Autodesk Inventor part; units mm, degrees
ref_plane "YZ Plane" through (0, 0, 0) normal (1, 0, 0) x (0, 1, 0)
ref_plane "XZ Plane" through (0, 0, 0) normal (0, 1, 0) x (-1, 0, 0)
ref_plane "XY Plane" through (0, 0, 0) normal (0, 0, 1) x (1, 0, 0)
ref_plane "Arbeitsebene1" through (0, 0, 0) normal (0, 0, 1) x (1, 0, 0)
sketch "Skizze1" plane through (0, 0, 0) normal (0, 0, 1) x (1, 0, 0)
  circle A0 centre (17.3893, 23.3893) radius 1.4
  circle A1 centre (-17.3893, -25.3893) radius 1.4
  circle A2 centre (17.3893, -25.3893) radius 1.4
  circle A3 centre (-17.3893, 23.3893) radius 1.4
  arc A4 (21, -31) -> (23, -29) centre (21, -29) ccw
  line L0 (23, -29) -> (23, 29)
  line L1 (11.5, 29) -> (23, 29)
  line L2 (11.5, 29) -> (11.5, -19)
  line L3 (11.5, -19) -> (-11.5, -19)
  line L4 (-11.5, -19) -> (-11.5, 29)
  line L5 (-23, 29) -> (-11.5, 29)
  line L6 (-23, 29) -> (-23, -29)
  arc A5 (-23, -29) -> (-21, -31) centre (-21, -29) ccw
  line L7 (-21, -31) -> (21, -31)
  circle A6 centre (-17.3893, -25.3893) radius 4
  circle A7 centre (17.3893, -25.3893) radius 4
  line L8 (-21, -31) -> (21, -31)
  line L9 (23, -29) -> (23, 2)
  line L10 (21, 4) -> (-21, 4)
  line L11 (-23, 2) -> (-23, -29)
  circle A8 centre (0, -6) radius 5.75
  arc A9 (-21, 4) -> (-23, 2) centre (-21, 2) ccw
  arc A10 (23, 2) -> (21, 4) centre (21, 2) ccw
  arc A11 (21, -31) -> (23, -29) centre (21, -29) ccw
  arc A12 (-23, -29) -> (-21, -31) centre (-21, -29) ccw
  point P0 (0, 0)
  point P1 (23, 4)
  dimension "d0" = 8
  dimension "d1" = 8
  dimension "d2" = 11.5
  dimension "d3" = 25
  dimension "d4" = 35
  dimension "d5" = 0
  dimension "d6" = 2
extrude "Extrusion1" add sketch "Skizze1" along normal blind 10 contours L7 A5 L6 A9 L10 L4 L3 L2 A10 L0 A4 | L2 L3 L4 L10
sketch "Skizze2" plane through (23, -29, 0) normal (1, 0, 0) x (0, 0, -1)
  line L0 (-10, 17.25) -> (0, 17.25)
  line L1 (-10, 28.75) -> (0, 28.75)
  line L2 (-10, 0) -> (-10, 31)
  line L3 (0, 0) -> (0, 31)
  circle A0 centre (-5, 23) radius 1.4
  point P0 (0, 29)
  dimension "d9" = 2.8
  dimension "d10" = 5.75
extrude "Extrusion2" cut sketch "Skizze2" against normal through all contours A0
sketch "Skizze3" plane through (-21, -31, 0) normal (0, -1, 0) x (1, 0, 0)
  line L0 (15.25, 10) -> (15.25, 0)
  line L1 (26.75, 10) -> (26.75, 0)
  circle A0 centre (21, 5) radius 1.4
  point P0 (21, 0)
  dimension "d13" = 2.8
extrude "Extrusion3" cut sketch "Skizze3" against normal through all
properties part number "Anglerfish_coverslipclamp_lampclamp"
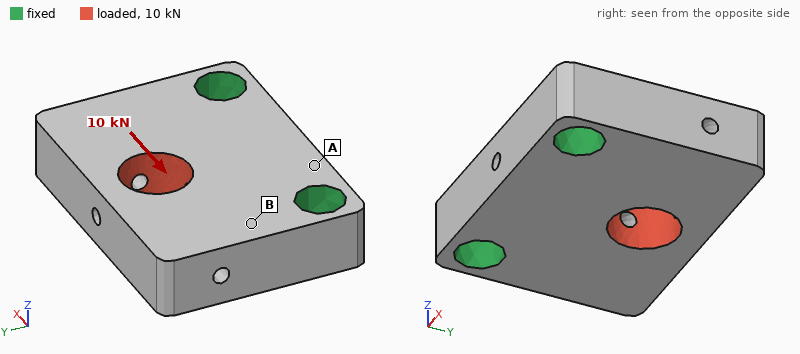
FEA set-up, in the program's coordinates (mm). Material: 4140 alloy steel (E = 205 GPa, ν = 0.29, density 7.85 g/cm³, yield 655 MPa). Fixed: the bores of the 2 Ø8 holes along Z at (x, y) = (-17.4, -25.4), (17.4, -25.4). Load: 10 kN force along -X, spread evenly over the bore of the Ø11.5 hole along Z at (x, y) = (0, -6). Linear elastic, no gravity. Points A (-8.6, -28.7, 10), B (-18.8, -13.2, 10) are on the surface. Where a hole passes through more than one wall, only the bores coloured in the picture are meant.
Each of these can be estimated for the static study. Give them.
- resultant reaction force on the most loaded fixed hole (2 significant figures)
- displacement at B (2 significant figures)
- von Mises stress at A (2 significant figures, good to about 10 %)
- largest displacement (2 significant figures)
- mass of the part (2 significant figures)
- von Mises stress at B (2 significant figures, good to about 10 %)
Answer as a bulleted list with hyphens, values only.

- 6.8 kN
- 4.3 µm
- 12 MPa
- 13 µm
- 110 g
- 32 MPa
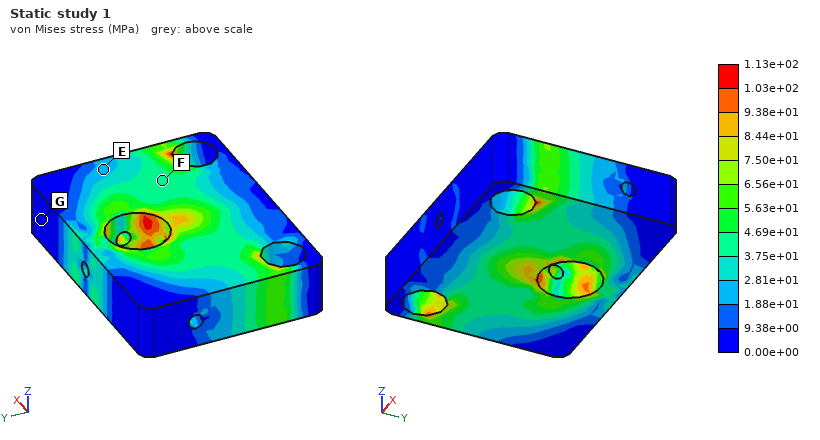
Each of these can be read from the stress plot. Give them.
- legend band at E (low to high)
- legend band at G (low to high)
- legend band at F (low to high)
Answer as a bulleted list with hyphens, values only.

- 1.88e+01 to 2.81e+01 MPa
- 0.00e+00 to 9.38e+00 MPa
- 3.75e+01 to 4.69e+01 MPa
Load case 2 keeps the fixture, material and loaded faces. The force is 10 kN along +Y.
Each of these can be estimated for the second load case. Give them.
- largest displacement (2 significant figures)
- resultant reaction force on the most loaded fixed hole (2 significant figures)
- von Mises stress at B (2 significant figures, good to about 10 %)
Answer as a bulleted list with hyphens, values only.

- 8.3 µm
- 5.4 kN
- 18 MPa
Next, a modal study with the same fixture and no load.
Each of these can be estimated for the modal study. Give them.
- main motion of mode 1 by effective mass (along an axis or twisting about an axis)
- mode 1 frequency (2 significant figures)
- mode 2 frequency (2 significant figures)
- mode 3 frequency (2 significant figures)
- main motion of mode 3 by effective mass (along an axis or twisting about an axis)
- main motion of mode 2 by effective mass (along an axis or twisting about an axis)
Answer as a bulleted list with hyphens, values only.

- along Z
- 9400 Hz
- 15 kHz
- 21 kHz
- along X
- twisting about Y
